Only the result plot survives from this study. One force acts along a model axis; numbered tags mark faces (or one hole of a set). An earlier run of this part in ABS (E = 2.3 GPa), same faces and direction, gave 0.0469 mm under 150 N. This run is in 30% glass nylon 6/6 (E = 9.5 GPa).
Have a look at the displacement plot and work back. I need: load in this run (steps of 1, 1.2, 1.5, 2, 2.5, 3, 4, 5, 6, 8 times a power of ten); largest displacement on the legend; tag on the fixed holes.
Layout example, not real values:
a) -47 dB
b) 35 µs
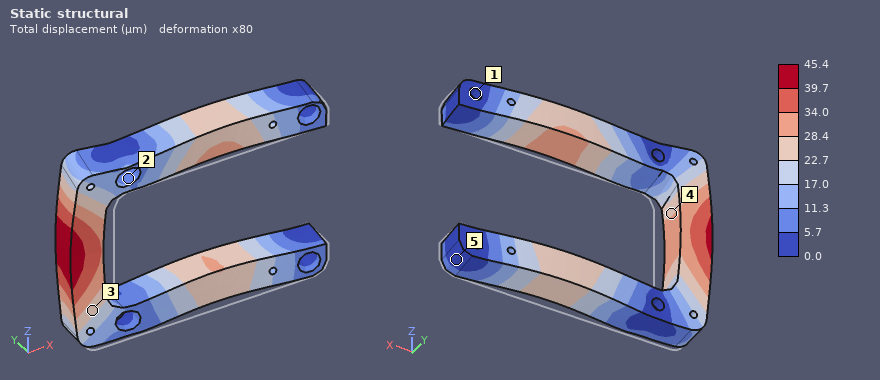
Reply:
a) 600 N
b) 45.4 µm
c) 1
